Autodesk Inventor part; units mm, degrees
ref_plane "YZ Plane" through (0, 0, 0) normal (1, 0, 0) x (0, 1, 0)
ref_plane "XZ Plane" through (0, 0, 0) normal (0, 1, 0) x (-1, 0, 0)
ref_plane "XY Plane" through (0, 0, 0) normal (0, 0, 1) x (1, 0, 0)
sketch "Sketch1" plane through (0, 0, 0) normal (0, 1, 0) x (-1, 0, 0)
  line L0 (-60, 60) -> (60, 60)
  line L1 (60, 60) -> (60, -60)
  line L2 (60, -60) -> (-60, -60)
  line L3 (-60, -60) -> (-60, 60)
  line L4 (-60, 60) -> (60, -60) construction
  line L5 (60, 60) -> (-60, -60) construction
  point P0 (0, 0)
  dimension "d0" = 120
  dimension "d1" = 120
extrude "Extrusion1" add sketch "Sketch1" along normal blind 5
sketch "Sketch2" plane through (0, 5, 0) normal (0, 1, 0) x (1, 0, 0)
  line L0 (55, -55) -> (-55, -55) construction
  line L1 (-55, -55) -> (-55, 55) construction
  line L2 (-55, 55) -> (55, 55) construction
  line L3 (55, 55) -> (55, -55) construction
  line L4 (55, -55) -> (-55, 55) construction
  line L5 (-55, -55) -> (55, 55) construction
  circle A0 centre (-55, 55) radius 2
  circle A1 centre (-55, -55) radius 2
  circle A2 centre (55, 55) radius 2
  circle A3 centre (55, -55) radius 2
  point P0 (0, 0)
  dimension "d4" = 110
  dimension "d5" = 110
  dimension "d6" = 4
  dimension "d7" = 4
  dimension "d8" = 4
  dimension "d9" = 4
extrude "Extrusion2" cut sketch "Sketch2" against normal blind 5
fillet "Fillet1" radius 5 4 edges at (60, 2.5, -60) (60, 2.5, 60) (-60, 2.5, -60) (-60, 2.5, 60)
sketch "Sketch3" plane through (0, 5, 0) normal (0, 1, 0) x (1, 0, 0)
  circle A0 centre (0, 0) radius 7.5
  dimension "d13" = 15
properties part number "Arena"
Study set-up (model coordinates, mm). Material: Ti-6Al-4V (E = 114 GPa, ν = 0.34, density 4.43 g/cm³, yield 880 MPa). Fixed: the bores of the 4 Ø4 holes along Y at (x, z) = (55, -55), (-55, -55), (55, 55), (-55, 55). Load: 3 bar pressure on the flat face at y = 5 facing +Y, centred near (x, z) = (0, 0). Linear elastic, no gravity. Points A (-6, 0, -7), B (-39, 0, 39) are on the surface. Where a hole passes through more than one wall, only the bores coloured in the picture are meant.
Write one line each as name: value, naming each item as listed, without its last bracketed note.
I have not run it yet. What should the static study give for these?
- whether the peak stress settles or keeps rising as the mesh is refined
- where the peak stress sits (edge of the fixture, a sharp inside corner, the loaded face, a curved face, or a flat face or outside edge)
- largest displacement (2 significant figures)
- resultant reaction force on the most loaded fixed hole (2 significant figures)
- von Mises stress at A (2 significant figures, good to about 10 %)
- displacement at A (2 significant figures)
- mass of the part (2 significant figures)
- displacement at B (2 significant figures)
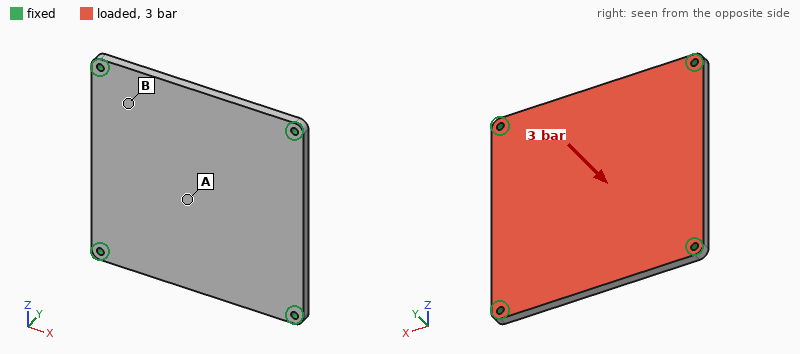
whether the peak stress settles or keeps rising as the mesh is refined: keeps rising
where the peak stress sits: edge of the fixture
largest displacement: 0.31 mm
resultant reaction force on the most loaded fixed hole: 1.1 kN
von Mises stress at A: 55 MPa
displacement at A: 0.31 mm
mass of the part: 320 g
displacement at B: 0.12 mm
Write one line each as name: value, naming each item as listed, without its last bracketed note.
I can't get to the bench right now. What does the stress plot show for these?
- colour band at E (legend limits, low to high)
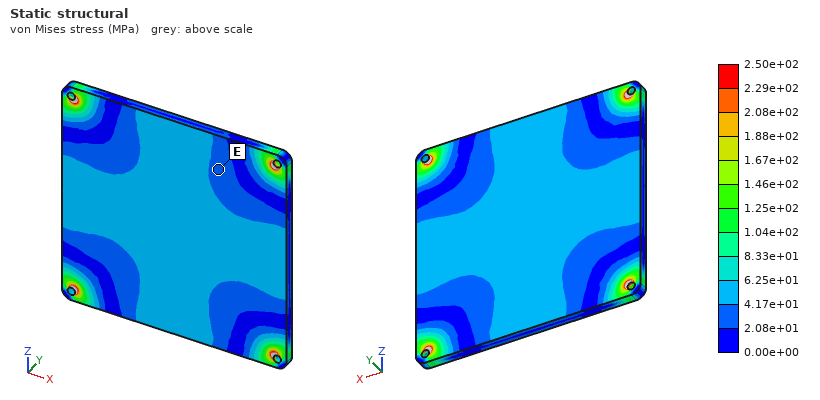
colour band at E: 2.08e+01 to 4.17e+01 MPa
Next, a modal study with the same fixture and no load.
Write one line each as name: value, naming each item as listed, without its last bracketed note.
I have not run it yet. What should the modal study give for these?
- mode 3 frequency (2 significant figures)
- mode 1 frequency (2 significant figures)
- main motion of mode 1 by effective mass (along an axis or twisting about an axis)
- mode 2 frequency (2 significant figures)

mode 3 frequency: 2300 Hz
mode 1 frequency: 1200 Hz
main motion of mode 1 by effective mass: along Y
mode 2 frequency: 2300 Hz
